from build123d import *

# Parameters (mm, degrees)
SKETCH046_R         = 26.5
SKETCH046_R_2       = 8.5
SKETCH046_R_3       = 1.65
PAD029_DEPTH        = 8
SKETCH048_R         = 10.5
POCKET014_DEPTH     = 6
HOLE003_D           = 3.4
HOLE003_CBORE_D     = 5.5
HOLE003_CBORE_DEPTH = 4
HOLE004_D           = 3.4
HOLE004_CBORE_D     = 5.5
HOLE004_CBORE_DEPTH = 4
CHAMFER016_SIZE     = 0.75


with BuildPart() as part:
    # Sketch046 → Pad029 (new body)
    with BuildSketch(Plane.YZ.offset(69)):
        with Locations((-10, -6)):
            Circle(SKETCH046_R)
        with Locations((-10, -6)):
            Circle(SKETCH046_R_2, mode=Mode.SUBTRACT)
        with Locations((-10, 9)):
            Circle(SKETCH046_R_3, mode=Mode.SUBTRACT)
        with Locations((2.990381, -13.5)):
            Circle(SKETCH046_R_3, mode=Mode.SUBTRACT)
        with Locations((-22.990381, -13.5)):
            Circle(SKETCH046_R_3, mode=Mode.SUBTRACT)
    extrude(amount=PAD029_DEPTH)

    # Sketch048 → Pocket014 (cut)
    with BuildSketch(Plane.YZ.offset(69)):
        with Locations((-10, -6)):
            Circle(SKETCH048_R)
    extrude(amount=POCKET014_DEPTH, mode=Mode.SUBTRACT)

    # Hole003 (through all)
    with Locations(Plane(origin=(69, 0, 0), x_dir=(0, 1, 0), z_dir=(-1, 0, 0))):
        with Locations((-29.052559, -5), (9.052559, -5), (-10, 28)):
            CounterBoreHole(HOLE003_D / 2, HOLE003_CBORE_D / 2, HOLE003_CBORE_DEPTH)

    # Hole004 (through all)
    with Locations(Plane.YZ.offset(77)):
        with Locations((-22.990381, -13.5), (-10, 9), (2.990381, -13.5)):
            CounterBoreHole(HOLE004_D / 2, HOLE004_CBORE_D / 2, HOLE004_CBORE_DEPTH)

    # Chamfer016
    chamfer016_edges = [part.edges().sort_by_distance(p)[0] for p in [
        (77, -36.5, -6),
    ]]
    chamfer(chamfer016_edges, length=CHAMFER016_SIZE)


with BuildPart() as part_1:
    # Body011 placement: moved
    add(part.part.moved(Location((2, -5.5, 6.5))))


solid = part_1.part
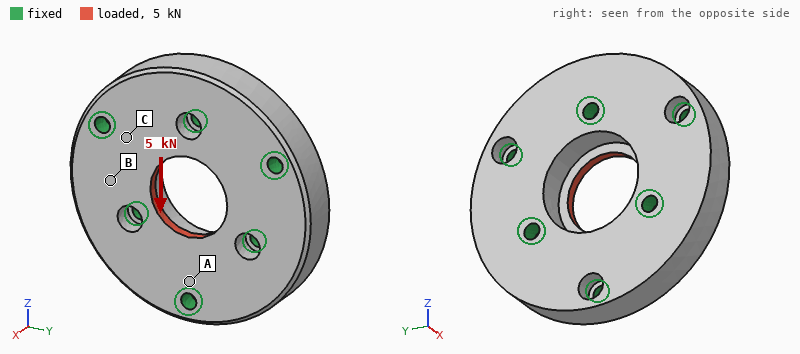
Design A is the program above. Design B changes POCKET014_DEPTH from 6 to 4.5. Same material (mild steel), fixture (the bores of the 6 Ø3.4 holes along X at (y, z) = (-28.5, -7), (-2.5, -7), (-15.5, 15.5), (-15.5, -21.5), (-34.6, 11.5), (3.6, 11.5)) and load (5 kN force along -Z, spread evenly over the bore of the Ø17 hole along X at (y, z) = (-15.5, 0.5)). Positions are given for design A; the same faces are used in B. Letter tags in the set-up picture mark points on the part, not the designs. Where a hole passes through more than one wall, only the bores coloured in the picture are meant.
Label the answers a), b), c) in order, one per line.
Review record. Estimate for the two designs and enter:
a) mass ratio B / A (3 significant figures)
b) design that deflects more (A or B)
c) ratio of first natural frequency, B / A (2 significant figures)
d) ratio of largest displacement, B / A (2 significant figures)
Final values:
a) 1.01
b) A
c) 1.0
d) 0.68
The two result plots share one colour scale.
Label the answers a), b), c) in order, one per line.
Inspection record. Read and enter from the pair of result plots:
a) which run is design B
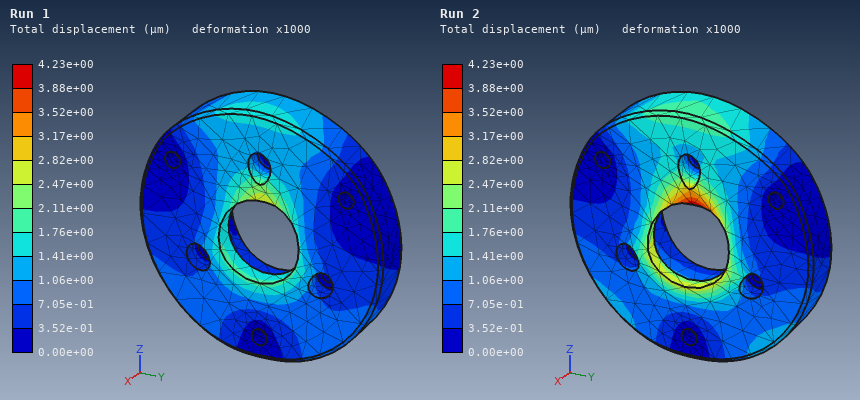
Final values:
a) Run 1
